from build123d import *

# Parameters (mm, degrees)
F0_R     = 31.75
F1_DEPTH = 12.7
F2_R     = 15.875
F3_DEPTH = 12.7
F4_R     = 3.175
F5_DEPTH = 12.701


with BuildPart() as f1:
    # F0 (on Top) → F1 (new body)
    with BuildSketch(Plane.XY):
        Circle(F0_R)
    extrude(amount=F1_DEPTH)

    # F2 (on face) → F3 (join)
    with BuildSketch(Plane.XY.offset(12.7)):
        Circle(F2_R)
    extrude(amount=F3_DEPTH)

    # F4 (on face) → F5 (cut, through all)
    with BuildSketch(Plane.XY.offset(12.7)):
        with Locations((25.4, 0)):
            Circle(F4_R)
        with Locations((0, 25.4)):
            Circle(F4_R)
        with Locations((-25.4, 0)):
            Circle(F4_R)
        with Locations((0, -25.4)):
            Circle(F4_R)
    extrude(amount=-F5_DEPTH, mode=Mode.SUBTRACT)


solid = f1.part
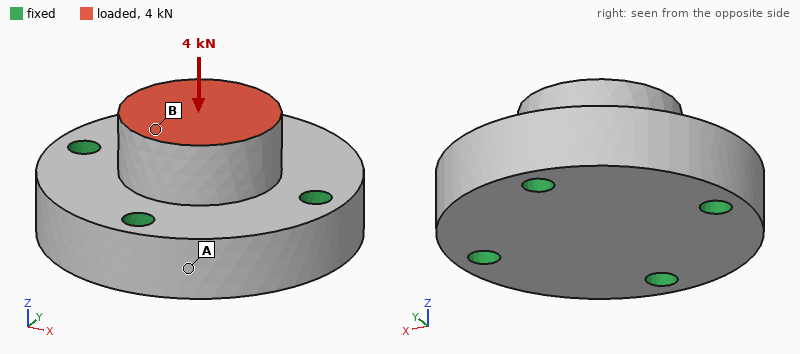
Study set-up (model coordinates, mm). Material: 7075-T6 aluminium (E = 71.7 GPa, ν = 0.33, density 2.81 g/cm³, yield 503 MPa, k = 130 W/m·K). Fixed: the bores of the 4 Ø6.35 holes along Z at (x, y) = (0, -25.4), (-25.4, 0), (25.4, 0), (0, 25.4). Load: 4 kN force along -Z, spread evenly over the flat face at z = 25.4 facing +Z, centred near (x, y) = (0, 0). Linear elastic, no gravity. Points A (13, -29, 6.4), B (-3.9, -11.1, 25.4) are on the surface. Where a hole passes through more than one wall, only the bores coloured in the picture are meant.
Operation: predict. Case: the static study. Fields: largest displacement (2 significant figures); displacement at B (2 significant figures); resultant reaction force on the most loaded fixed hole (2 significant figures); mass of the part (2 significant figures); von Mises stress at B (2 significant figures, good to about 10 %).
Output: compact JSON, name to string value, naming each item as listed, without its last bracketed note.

{"largest displacement": "3.5 µm", "displacement at B": "3.5 µm", "resultant reaction force on the most loaded fixed hole": "1.0 kN", "mass of the part": "140 g", "von Mises stress at B": "5.1 MPa"}
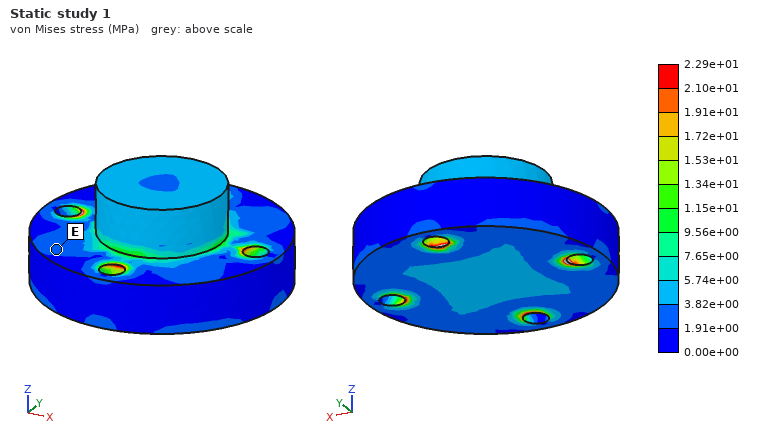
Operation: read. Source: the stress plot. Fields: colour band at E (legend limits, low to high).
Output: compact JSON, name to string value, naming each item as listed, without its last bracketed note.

{"colour band at E": "1.91e+00 to 3.82e+00 MPa"}
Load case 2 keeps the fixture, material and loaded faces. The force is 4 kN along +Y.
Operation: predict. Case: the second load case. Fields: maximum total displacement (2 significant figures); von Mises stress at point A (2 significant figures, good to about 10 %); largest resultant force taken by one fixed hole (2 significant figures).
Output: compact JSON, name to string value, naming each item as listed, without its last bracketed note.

{"maximum total displacement": "10.0 µm", "von Mises stress at point A": "3.8 MPa", "largest resultant force taken by one fixed hole": "2.0 kN"}
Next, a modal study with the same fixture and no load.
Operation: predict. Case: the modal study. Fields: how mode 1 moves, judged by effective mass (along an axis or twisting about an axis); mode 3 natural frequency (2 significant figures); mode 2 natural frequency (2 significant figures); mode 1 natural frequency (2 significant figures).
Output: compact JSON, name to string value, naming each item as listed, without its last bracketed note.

{"how mode 1 moves, judged by effective mass": "along Z", "mode 3 natural frequency": "24 kHz", "mode 2 natural frequency": "24 kHz", "mode 1 natural frequency": "23 kHz"}
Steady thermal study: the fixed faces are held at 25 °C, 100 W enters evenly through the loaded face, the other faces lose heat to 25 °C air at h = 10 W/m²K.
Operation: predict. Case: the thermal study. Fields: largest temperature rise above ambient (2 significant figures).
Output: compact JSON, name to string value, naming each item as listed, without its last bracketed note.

{"largest temperature rise above ambient": "24 K"}
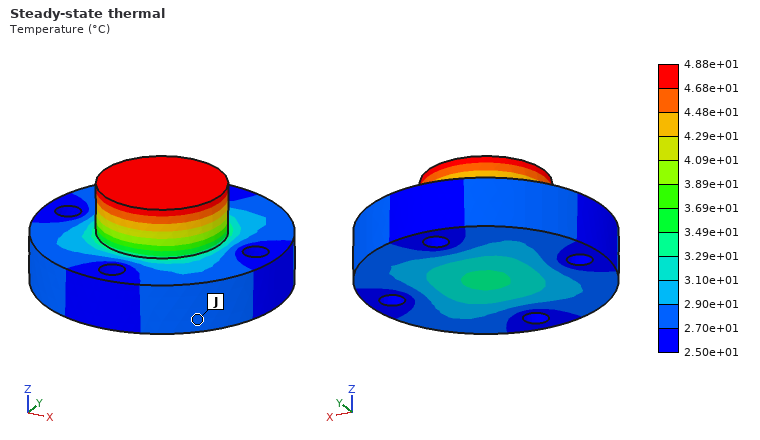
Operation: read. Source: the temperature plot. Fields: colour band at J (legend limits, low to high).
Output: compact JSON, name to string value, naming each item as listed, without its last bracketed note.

{"colour band at J": "2.70e+01 to 2.90e+01 °C"}
